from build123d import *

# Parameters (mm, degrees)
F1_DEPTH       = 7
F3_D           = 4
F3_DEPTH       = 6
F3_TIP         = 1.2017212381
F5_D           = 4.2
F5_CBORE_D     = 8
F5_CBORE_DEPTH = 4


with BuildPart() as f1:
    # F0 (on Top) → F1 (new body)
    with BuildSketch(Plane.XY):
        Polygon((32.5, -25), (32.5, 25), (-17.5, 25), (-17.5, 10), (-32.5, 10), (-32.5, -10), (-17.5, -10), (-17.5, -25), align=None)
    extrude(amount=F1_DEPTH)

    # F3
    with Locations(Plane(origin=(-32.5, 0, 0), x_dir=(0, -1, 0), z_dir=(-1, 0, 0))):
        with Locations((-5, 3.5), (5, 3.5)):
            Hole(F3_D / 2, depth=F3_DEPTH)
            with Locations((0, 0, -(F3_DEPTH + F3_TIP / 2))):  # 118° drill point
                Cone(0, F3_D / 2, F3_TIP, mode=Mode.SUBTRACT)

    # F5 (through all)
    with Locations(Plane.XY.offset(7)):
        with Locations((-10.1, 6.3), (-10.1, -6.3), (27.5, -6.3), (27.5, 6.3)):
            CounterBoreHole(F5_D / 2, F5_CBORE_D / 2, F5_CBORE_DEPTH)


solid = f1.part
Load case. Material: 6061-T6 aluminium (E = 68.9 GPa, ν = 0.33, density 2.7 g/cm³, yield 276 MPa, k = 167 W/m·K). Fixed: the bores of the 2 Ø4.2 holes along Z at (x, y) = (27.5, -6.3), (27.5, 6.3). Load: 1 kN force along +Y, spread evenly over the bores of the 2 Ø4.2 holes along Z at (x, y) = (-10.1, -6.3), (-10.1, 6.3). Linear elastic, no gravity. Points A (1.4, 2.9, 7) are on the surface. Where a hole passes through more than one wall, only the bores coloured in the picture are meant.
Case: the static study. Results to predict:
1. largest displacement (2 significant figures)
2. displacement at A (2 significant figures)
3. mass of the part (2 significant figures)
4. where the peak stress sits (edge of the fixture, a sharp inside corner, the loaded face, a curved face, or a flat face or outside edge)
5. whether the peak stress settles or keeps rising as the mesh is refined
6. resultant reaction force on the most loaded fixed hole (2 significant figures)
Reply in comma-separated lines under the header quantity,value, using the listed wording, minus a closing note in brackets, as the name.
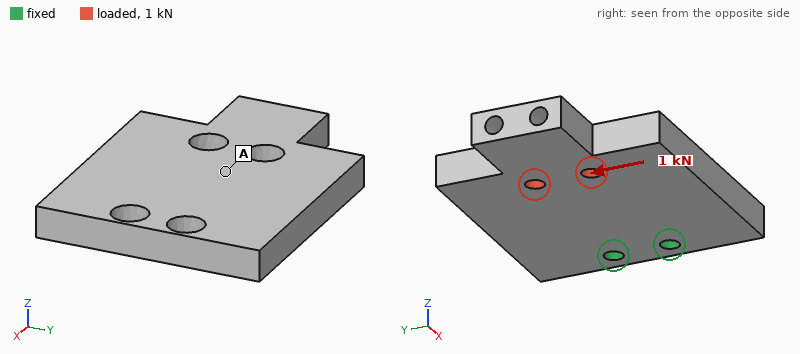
quantity,value
largest displacement,80 µm
displacement at A,30 µm
mass of the part,50 g
where the peak stress sits,edge of the fixture
whether the peak stress settles or keeps rising as the mesh is refined,keeps rising
resultant reaction force on the most loaded fixed hole,2.3 kN
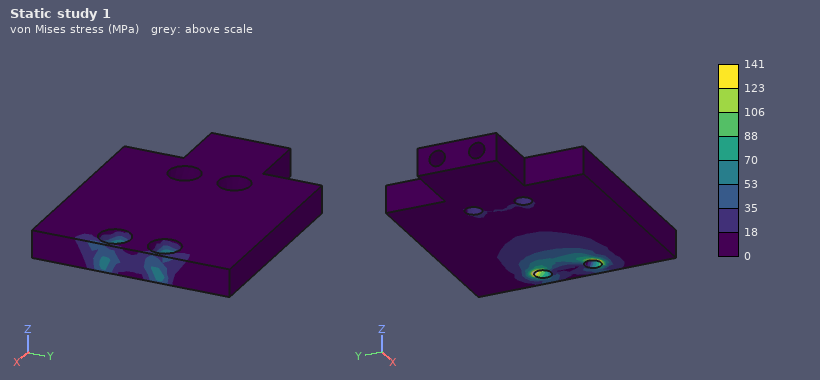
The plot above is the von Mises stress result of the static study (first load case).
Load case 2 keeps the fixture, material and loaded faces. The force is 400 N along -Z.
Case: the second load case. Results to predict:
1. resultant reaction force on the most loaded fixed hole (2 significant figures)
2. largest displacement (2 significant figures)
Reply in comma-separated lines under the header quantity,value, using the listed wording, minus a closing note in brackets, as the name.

quantity,value
resultant reaction force on the most loaded fixed hole,250 N
largest displacement,0.35 mm
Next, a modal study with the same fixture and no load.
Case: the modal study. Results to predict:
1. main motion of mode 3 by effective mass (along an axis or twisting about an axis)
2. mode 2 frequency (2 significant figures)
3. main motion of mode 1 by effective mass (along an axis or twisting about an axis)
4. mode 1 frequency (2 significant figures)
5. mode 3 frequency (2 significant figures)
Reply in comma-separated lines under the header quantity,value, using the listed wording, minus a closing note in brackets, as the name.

quantity,value
main motion of mode 3 by effective mass,along Y
mode 2 frequency,3600 Hz
main motion of mode 1 by effective mass,along Z
mode 1 frequency,1300 Hz
mode 3 frequency,4100 Hz
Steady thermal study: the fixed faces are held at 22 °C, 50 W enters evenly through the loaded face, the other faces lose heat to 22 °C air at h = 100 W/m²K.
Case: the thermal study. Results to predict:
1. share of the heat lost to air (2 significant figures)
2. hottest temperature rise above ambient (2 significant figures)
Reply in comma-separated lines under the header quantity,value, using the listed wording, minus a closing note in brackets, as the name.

quantity,value
share of the heat lost to air,32 %
hottest temperature rise above ambient,42 K
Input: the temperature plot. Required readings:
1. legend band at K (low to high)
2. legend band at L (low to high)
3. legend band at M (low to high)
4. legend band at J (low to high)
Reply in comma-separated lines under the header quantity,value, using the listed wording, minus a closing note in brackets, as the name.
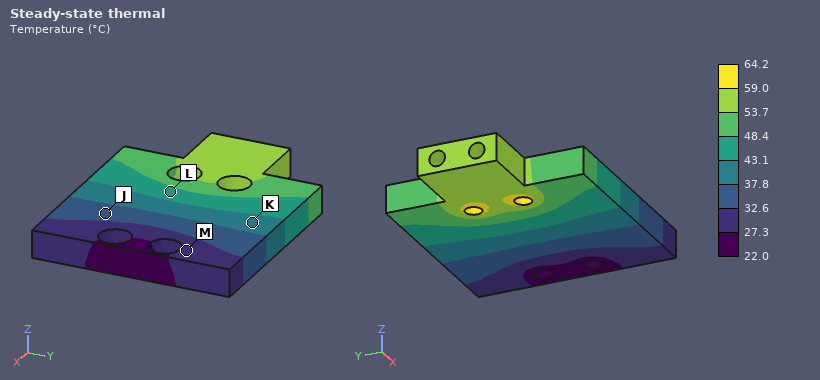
quantity,value
legend band at K,37.8 to 43.1 °C
legend band at L,43.1 to 48.4 °C
legend band at M,27.3 to 32.6 °C
legend band at J,32.6 to 37.8 °C
